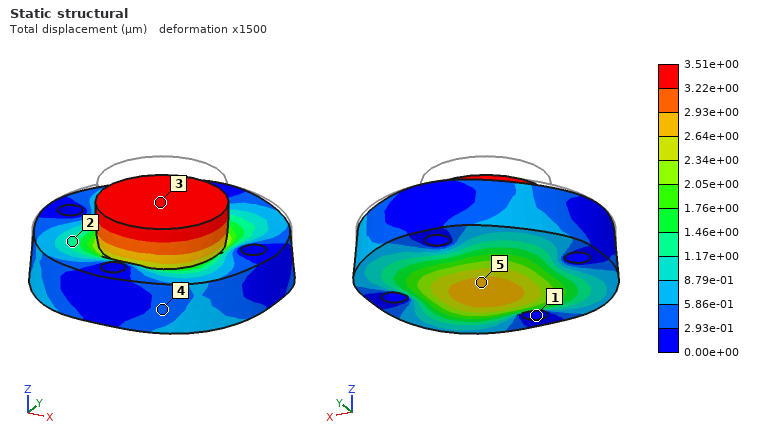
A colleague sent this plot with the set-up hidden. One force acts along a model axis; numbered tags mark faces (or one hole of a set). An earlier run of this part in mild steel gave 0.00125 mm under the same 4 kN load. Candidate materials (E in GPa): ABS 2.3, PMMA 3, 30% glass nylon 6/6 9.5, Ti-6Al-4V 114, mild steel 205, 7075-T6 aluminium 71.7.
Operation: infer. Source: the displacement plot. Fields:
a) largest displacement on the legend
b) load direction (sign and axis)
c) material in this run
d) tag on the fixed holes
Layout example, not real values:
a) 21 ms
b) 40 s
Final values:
a) 3.51e+00 µm
b) -Z
c) 7075-T6 aluminium
d) 1
